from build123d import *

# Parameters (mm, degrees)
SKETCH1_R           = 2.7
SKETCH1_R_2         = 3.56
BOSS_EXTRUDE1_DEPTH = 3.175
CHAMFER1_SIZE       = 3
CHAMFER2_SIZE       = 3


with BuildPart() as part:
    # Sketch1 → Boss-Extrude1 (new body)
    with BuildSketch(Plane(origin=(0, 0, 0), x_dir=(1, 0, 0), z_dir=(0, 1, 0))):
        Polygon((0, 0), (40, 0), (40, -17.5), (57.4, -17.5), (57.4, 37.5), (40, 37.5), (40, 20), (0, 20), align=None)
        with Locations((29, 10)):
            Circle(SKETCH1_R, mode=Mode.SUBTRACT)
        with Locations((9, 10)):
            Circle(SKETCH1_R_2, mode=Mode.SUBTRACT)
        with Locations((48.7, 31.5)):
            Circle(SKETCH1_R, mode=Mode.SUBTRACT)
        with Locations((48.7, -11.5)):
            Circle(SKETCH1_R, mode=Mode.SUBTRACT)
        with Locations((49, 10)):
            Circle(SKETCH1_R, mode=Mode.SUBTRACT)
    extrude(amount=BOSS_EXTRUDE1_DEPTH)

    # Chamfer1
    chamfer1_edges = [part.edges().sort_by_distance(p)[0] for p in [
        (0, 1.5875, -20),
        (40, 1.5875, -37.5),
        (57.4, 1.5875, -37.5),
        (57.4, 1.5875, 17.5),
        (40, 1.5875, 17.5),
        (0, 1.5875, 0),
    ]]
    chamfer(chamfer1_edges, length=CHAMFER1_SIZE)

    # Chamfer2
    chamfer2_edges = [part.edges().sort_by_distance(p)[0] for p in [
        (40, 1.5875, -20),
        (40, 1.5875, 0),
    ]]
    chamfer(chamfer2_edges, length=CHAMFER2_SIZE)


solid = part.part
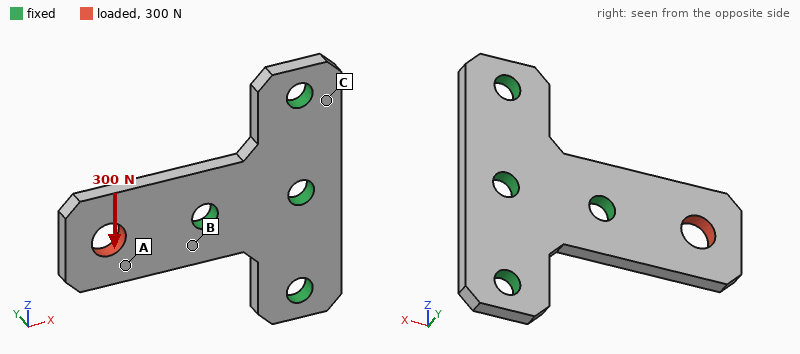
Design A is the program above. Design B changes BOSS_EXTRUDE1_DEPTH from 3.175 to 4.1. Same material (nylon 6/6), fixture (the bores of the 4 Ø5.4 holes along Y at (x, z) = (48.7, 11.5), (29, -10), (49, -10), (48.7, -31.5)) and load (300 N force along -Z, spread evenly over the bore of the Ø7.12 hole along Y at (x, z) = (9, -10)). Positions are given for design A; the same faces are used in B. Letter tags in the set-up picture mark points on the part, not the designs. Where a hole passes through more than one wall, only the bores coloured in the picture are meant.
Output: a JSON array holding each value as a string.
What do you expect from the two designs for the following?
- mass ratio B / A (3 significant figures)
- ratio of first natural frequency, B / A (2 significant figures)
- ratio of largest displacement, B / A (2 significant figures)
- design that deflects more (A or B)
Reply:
["1.29", "1.3", "0.77", "A"]
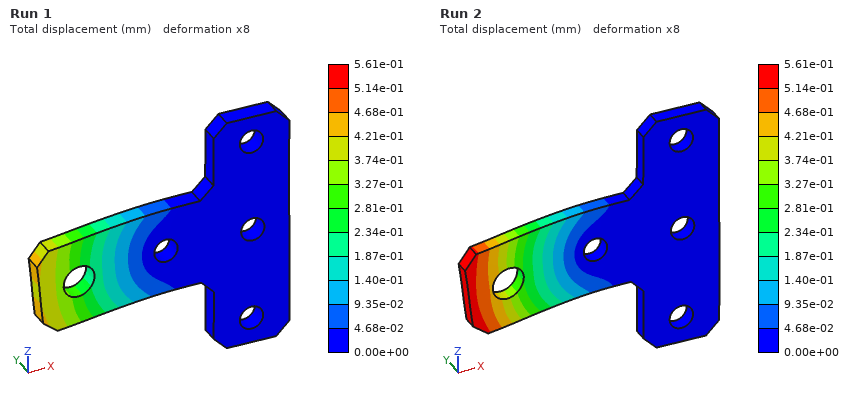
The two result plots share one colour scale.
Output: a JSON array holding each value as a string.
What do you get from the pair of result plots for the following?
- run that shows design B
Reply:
["Run 1"]
